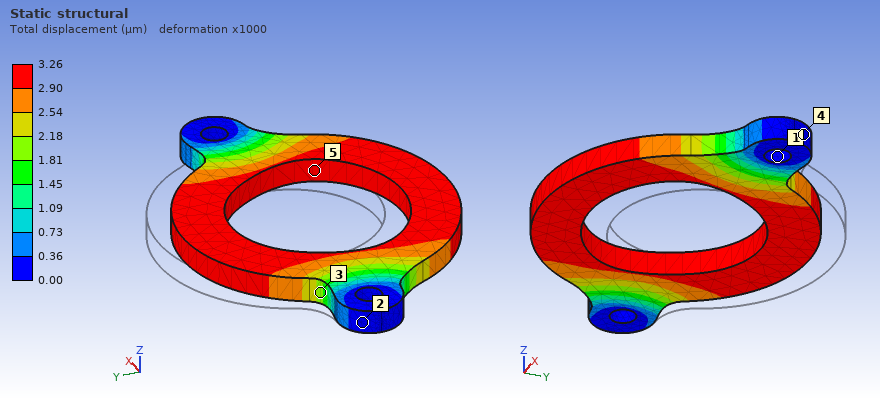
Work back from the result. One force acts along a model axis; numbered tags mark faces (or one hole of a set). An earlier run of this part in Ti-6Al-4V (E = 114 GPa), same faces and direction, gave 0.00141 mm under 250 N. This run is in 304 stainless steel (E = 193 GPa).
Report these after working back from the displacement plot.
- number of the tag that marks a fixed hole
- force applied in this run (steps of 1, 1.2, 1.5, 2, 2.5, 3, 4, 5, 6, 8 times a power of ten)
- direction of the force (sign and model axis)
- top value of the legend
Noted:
1
1 kN
-Y
3.26 µm
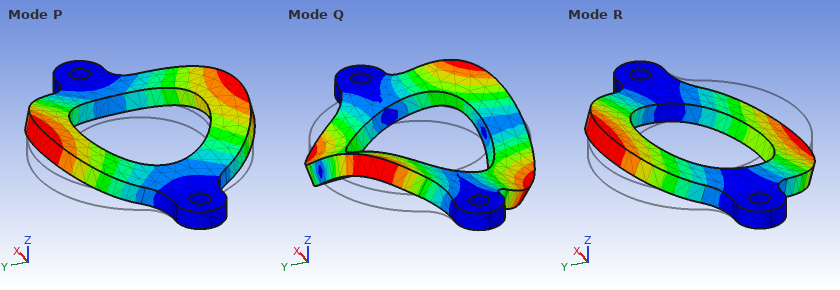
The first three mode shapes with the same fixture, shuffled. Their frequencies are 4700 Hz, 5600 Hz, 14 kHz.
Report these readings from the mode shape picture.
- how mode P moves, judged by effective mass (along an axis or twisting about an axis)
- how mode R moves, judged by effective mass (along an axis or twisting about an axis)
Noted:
along Z
twisting about X
